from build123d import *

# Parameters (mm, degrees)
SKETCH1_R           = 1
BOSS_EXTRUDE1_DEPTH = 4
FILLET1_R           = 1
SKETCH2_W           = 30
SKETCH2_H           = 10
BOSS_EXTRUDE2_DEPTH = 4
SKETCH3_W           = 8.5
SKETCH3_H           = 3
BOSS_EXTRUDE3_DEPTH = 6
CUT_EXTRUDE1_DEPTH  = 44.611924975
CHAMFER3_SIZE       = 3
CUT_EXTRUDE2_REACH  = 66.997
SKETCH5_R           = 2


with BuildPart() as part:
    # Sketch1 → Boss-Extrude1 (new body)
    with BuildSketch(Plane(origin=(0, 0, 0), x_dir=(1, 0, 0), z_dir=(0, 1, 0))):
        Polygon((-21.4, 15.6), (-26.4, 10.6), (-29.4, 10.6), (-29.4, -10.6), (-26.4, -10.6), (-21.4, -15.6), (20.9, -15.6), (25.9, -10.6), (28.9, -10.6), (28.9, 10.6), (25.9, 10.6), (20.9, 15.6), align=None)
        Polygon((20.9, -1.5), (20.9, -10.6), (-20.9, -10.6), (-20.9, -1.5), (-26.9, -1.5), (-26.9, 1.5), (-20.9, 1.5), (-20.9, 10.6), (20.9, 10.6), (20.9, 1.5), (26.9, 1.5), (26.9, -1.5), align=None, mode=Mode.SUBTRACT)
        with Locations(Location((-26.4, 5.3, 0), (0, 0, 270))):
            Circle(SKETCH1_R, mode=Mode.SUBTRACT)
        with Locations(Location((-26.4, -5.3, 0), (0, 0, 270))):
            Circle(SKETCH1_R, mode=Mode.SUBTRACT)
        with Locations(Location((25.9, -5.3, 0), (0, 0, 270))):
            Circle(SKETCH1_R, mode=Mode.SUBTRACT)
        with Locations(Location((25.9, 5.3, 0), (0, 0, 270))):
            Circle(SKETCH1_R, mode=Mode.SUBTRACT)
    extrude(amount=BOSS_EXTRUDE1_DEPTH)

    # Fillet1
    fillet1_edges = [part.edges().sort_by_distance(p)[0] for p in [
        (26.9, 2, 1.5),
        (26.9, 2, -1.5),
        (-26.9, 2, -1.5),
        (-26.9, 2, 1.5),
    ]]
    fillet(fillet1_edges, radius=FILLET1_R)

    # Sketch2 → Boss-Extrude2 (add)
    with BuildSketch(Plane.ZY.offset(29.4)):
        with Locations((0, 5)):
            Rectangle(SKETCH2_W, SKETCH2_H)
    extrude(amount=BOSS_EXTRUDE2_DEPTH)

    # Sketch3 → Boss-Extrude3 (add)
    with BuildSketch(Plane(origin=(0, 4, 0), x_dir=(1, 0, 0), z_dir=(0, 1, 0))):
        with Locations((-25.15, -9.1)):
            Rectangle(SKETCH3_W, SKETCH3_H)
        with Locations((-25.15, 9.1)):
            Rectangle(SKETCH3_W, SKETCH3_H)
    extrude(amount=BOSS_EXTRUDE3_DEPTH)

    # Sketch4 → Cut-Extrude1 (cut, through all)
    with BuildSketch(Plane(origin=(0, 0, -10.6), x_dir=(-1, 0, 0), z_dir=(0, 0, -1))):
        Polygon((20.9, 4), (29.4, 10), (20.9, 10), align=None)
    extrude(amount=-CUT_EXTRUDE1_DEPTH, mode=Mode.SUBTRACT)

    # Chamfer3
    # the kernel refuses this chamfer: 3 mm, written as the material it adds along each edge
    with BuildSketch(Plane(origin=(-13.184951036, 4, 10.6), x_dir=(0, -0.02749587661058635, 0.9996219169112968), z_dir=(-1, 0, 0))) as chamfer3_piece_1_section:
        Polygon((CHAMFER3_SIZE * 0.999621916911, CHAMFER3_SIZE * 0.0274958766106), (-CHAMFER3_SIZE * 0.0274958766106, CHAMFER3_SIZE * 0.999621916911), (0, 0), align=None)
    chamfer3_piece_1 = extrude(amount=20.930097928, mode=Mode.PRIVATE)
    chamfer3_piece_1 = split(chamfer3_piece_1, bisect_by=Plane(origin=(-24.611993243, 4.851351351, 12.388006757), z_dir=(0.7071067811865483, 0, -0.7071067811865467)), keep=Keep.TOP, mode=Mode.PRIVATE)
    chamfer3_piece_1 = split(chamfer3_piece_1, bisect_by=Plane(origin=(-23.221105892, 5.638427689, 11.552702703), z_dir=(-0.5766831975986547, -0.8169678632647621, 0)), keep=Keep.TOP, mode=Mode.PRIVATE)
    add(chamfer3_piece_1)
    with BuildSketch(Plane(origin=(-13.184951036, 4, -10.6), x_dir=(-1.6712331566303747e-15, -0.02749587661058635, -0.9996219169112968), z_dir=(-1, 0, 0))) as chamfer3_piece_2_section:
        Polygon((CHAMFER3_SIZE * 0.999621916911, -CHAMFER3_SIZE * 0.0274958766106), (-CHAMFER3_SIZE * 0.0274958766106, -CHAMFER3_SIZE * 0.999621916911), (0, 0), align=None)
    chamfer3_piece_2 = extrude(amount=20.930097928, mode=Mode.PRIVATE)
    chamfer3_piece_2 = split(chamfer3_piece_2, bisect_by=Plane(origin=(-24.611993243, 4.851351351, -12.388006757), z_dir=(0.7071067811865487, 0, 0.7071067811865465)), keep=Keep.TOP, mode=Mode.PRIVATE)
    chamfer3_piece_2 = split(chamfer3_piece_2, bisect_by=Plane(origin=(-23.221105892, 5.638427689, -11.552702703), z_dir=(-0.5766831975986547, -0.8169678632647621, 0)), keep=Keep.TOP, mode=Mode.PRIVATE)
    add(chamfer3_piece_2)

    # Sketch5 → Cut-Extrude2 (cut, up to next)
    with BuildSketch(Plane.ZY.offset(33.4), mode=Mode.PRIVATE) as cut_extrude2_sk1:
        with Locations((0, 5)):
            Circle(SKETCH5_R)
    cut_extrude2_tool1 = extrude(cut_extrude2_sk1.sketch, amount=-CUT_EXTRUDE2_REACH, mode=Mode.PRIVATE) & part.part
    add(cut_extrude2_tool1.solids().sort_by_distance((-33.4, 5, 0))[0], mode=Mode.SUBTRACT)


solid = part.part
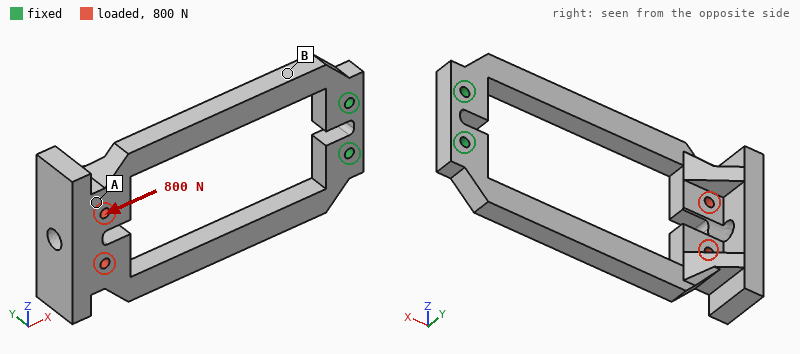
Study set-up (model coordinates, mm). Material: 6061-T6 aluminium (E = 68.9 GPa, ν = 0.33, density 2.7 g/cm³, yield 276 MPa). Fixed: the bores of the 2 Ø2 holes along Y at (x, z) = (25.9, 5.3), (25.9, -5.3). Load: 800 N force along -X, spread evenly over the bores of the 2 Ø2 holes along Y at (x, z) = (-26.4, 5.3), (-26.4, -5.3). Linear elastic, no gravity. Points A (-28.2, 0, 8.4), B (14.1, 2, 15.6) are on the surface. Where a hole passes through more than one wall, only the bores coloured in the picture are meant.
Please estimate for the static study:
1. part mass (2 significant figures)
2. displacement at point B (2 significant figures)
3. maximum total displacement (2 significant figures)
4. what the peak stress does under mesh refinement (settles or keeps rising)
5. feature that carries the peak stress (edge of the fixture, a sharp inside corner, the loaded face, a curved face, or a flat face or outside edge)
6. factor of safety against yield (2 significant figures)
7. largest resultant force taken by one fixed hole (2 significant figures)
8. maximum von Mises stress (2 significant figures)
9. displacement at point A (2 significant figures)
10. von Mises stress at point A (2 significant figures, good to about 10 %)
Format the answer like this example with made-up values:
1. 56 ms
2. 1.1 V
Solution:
1. 12 g
2. 45 µm
3. 69 µm
4. settles
5. a curved face
6. 1.1
7. 470 N
8. 260 MPa
9. 52 µm
10. 39 MPa
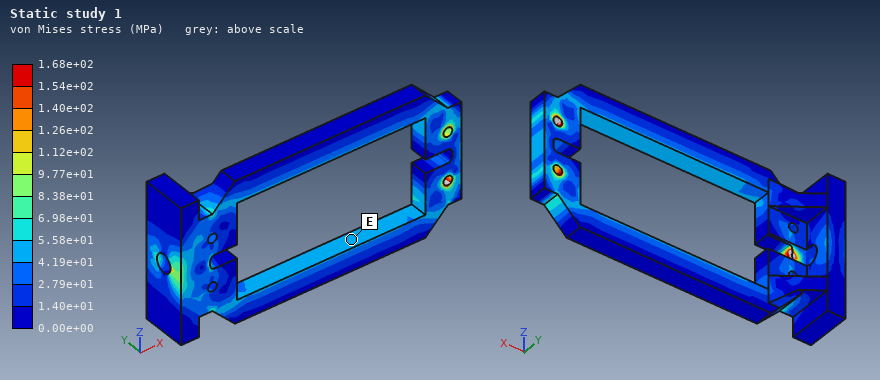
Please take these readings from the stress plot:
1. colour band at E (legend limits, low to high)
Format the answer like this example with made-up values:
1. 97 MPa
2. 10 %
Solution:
1. 4.19e+01 to 5.58e+01 MPa
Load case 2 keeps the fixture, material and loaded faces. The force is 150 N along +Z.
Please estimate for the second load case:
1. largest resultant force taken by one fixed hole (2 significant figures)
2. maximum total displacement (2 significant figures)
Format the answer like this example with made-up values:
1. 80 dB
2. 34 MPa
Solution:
1. 350 N
2. 0.52 mm
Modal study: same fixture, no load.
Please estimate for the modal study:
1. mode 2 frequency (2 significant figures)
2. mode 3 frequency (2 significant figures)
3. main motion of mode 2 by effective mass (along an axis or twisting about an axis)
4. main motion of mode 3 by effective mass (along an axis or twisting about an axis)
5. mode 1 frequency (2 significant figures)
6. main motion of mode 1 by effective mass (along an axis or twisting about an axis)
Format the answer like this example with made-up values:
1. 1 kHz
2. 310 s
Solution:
1. 1000 Hz
2. 1800 Hz
3. along Z
4. twisting about X
5. 470 Hz
6. along Y
